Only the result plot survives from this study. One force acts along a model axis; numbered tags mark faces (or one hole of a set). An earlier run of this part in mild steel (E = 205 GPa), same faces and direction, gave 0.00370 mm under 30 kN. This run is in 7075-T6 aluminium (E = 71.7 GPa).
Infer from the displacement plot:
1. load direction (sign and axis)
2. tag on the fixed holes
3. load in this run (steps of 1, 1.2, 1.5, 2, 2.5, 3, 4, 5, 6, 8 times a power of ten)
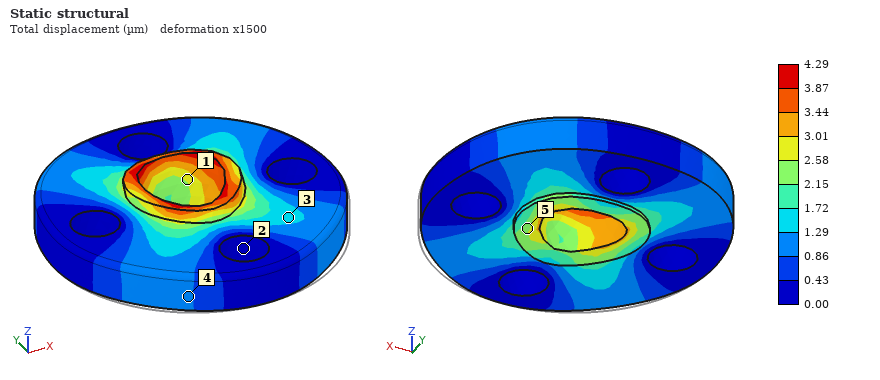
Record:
+Y
2
12 kN
